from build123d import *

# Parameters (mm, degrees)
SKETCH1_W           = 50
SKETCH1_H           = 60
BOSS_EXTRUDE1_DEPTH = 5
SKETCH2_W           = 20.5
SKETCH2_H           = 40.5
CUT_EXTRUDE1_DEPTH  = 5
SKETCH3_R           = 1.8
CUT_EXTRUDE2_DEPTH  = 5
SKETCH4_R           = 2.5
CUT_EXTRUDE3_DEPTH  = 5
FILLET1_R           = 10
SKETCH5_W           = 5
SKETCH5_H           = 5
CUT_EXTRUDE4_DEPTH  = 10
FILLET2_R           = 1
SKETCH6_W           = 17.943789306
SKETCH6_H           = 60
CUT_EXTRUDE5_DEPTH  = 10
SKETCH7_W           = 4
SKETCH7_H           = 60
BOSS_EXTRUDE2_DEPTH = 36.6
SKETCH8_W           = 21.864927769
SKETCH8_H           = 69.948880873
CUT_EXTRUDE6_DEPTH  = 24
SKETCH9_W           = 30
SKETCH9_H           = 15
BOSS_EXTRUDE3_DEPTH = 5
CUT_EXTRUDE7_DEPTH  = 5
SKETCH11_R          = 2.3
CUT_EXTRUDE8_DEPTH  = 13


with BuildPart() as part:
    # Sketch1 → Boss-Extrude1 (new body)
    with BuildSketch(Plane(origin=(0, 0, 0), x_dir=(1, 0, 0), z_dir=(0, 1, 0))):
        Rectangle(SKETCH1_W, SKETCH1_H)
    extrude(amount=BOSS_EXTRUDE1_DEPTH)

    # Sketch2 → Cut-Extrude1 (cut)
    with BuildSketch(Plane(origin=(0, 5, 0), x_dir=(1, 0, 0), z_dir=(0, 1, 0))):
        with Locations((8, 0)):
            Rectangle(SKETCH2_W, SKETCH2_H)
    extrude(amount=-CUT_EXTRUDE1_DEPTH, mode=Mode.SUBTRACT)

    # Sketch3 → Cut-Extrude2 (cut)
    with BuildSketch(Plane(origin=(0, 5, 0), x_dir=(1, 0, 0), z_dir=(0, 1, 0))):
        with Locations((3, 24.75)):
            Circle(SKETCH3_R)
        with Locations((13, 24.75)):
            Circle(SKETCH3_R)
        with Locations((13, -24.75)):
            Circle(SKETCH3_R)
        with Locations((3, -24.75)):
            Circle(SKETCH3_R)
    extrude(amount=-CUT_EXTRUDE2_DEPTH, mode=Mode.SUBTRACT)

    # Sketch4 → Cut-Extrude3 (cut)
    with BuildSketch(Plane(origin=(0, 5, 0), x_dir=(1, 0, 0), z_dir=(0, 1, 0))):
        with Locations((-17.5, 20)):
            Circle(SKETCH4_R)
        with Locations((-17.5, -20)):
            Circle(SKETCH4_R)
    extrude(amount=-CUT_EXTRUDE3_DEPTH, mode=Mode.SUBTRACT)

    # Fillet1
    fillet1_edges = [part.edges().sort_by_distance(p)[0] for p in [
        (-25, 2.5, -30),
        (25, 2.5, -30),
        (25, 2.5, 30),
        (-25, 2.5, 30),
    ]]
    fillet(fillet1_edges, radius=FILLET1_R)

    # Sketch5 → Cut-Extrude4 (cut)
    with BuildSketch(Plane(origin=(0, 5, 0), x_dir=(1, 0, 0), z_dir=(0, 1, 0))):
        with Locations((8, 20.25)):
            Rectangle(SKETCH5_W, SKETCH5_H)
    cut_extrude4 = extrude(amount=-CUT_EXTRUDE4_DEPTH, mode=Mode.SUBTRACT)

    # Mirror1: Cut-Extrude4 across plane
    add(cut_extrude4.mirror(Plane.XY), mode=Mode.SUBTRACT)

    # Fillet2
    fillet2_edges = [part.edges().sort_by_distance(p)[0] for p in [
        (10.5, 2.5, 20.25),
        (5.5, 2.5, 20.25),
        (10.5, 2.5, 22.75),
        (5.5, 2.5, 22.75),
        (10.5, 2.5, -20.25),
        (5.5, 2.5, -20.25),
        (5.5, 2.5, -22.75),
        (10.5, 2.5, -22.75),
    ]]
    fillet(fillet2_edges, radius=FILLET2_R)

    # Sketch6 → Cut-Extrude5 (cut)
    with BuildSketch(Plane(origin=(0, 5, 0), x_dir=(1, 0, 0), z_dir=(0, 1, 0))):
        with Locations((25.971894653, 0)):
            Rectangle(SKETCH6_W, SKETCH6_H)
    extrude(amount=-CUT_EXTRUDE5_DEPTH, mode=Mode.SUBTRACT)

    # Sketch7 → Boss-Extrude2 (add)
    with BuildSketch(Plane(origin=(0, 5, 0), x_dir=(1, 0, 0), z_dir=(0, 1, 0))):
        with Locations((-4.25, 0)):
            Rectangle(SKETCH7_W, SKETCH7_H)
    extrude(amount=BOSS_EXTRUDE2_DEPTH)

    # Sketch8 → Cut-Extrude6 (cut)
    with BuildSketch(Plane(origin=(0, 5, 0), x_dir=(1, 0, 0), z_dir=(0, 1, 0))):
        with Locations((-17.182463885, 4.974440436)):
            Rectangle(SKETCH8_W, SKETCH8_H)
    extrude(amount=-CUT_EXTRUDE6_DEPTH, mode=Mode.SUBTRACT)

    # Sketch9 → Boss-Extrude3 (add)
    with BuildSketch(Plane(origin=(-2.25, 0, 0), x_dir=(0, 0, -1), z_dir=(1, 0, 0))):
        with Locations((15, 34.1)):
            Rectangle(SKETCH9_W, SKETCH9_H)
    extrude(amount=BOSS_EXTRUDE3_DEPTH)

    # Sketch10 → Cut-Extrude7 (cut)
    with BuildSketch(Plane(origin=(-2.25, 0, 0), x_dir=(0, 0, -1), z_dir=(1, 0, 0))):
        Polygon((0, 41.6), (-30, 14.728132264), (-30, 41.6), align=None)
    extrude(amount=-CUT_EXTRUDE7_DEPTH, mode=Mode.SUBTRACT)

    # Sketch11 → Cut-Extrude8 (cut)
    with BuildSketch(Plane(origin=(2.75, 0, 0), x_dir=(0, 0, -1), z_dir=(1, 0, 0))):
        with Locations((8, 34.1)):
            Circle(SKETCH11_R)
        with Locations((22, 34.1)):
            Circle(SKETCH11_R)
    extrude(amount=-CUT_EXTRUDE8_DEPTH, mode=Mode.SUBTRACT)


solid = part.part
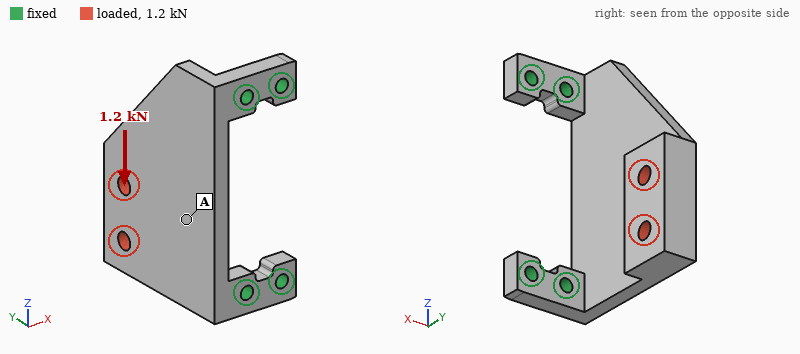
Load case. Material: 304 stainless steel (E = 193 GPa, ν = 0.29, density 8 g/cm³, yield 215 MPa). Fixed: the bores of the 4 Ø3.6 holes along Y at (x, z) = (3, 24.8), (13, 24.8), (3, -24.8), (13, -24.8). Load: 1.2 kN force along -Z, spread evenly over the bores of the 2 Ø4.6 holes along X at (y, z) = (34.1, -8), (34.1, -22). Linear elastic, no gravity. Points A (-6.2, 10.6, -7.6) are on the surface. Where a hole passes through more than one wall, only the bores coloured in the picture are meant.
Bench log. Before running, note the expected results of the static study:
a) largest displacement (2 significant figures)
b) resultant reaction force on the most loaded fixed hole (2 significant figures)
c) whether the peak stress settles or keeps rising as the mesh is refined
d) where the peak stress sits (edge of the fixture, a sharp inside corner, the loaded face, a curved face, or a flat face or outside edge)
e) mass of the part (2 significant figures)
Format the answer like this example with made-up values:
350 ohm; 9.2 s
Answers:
32 µm; 1.1 kN; keeps rising; edge of the fixture; 95 g
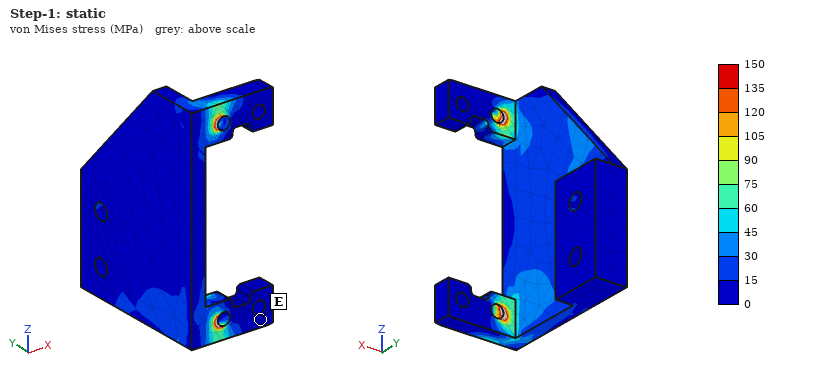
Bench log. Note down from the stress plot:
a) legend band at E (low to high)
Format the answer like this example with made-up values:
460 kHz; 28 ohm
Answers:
0 to 15 MPa
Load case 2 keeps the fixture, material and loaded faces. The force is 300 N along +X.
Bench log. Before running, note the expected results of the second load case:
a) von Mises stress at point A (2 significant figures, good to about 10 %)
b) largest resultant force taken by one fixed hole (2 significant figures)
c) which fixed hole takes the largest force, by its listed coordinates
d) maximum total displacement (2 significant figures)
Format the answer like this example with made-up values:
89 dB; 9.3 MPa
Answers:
29 MPa; 240 N; (3, -24.8); 0.18 mm
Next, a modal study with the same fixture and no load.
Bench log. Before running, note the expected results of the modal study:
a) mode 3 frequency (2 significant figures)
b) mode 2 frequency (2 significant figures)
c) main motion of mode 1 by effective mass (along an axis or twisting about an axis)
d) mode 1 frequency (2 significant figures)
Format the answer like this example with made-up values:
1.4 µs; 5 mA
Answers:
6700 Hz; 4200 Hz; along X; 1200 Hz
